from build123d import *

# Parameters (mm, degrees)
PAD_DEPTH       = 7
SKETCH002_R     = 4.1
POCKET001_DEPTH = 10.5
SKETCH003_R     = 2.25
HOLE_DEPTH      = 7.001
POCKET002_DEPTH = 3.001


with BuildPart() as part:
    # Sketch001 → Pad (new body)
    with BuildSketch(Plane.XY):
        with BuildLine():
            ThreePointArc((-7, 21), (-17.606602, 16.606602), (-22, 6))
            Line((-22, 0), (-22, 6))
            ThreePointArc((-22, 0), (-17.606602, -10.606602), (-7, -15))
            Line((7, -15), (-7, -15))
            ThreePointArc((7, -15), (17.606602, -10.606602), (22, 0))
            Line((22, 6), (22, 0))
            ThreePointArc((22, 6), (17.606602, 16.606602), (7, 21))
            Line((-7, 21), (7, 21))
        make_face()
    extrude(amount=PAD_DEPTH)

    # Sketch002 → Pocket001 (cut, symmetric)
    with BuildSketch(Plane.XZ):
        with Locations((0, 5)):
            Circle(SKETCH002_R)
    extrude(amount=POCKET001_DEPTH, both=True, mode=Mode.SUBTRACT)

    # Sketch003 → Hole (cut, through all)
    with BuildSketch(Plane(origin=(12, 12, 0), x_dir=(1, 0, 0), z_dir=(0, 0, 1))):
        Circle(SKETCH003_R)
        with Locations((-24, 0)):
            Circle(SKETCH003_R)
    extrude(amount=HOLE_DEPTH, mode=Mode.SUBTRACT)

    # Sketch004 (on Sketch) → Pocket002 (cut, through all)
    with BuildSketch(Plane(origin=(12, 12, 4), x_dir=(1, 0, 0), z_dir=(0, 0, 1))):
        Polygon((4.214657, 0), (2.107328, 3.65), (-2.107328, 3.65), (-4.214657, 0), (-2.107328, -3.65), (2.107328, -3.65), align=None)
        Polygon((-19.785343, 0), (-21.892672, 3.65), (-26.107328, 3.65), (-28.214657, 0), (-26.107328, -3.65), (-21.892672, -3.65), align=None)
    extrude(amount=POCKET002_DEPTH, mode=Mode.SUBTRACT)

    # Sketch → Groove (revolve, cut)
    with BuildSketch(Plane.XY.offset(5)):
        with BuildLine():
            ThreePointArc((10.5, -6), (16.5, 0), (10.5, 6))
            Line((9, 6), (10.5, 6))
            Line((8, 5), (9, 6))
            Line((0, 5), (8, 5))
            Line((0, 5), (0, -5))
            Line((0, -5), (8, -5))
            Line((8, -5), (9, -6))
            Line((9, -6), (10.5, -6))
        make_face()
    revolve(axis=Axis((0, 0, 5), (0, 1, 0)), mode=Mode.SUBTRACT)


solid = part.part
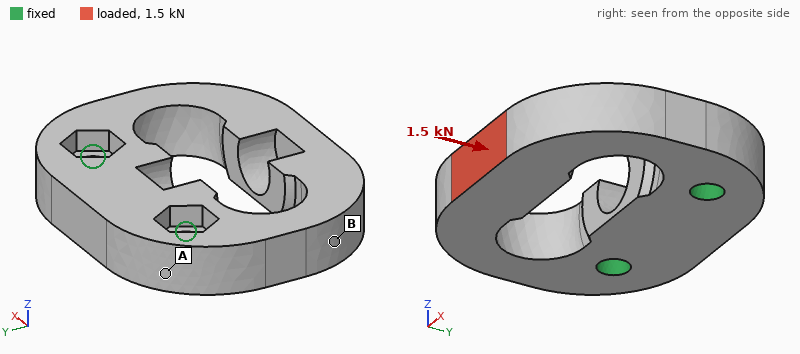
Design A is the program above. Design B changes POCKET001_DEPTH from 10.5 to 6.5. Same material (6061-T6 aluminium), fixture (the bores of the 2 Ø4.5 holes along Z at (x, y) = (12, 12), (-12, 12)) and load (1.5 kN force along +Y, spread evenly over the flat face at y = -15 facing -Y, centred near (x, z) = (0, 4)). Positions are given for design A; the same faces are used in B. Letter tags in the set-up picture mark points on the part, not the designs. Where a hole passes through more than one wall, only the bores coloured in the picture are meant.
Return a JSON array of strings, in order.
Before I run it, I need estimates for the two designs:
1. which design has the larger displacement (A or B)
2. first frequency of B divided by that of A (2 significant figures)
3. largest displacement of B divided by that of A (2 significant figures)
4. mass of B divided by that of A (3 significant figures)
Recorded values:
["A", "0.98", "0.75", "1.05"]
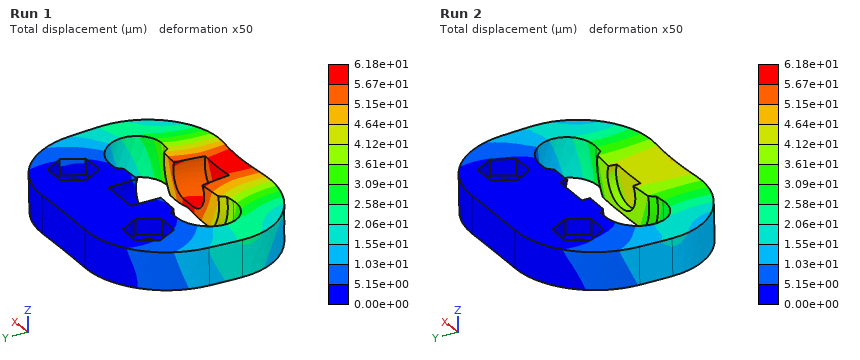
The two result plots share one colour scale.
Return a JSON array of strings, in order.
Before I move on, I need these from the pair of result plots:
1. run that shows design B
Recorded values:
["Run 2"]
